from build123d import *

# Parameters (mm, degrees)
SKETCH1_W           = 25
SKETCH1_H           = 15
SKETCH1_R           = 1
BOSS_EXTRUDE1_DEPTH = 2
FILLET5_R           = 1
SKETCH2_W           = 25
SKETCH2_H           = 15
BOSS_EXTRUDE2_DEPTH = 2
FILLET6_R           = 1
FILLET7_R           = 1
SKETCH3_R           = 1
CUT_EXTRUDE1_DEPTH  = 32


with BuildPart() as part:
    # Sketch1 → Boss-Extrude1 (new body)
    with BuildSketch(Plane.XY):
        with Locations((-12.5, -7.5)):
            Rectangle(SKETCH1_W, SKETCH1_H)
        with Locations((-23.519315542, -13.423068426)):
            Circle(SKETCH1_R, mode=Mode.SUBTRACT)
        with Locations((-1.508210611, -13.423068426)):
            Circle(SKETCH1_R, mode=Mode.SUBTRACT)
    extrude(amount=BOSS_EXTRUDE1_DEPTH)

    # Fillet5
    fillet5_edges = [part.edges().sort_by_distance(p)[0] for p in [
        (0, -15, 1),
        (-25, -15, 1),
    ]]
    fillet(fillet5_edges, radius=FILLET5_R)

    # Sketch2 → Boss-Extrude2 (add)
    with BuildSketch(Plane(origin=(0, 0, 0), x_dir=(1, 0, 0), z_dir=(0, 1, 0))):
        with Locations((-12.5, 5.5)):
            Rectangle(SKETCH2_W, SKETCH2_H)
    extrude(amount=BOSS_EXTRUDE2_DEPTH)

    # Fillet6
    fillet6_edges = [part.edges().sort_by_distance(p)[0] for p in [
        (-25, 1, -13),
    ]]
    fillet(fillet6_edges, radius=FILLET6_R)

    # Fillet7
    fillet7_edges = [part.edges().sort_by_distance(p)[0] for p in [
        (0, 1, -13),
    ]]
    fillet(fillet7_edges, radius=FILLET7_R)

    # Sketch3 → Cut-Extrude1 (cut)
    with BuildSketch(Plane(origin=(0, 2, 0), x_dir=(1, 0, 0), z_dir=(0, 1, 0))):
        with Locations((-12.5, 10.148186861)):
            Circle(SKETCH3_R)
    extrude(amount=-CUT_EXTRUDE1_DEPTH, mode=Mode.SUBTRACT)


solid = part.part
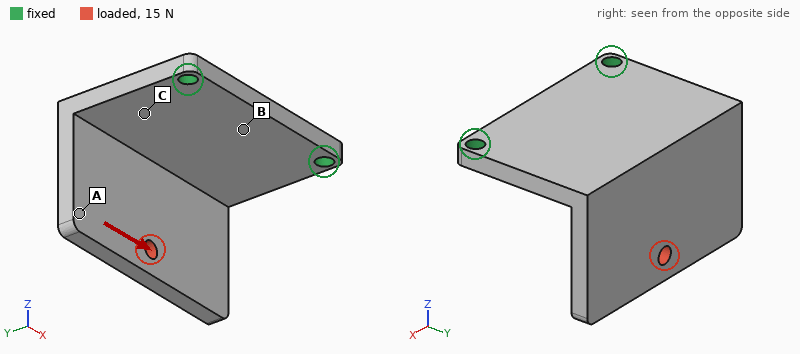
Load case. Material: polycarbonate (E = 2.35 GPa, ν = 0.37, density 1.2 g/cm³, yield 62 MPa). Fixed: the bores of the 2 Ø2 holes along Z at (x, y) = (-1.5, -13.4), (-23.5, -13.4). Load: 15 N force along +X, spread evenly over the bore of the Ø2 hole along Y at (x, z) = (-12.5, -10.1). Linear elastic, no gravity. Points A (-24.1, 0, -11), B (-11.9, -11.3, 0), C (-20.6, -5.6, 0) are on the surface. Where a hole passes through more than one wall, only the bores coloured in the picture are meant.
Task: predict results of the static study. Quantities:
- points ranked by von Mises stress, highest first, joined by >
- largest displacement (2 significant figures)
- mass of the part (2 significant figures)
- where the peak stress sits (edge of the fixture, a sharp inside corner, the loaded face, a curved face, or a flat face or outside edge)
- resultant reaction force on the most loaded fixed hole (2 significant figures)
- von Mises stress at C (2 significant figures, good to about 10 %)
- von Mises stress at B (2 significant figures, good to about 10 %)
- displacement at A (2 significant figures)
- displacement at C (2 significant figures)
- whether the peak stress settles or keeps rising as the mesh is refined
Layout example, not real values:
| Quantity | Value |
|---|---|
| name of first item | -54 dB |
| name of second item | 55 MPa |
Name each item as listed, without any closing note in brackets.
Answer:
| Quantity | Value |
|---|---|
| points ranked by von Mises stress, highest first, joined by > | C > B > A |
| largest displacement | 0.37 mm |
| mass of the part | 1.8 g |
| where the peak stress sits | edge of the fixture |
| resultant reaction force on the most loaded fixed hole | 15 N |
| von Mises stress at C | 5.7 MPa |
| von Mises stress at B | 3.2 MPa |
| displacement at A | 0.33 mm |
| displacement at C | 0.073 mm |
| whether the peak stress settles or keeps rising as the mesh is refined | keeps rising |
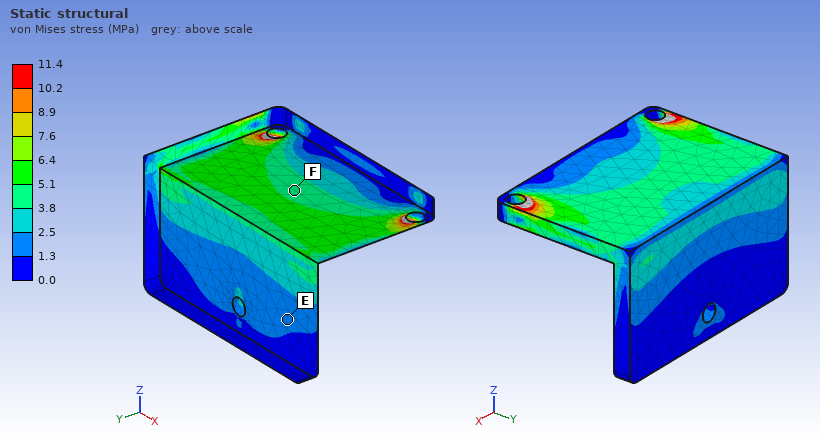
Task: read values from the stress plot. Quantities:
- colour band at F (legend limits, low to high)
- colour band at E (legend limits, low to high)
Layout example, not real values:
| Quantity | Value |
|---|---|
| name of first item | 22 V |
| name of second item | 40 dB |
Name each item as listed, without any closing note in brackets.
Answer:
| Quantity | Value |
|---|---|
| colour band at F | 3.8 to 5.1 MPa |
| colour band at E | 1.3 to 2.5 MPa |
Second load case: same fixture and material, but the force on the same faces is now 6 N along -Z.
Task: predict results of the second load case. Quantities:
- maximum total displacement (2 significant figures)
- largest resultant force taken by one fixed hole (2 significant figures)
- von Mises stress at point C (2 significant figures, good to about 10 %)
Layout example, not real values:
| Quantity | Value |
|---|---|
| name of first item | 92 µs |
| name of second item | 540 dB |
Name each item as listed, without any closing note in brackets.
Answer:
| Quantity | Value |
|---|---|
| maximum total displacement | 0.40 mm |
| largest resultant force taken by one fixed hole | 3.0 N |
| von Mises stress at point C | 2.6 MPa |
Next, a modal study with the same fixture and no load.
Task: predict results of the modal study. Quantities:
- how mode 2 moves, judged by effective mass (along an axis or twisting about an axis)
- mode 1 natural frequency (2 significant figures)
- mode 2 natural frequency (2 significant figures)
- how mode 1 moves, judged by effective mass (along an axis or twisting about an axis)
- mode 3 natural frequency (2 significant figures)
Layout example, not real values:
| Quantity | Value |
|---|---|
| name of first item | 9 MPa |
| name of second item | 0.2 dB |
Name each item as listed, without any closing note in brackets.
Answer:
| Quantity | Value |
|---|---|
| how mode 2 moves, judged by effective mass | along X |
| mode 1 natural frequency | 640 Hz |
| mode 2 natural frequency | 1400 Hz |
| how mode 1 moves, judged by effective mass | along Z |
| mode 3 natural frequency | 2000 Hz |
